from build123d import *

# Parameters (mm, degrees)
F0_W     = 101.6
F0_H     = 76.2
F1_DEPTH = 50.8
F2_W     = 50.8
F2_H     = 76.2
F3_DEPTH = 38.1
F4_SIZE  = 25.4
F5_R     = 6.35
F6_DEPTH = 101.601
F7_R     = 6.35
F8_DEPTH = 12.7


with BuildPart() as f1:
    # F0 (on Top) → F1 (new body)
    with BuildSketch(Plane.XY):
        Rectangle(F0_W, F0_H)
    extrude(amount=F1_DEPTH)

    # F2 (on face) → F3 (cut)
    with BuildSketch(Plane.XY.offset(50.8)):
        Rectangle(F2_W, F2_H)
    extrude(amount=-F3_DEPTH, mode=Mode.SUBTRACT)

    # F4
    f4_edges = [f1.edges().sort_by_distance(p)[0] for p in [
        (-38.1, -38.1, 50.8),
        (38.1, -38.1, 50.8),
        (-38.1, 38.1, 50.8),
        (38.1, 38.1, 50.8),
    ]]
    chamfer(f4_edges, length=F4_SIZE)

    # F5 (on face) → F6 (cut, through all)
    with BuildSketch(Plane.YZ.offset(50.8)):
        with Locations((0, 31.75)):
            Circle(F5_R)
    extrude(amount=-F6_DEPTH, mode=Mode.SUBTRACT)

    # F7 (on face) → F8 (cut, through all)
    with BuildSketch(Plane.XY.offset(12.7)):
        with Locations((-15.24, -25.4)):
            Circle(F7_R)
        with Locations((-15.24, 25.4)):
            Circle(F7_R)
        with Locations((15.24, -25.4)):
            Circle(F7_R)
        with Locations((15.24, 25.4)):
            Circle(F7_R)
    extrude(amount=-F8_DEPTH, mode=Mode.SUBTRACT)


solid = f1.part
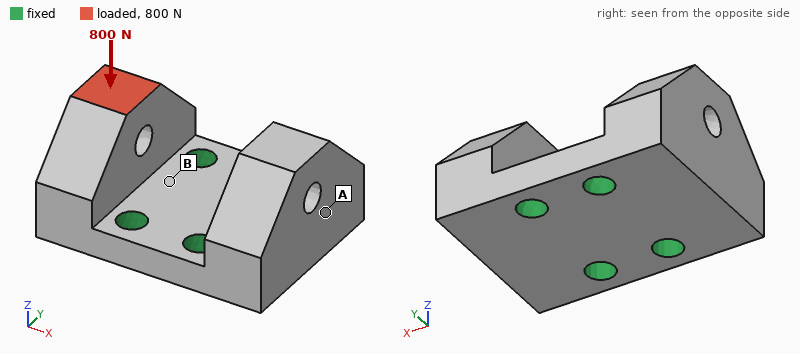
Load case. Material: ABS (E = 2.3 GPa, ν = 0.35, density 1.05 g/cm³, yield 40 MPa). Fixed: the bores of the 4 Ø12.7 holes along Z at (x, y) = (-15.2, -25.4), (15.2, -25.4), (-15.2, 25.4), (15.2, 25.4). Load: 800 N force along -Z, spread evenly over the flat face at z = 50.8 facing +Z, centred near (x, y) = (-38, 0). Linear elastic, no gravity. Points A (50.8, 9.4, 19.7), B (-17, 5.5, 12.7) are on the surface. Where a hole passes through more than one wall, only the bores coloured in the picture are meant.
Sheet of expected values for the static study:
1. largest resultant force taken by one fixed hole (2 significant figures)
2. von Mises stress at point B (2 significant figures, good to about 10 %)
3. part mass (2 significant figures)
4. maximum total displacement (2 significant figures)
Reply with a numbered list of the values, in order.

1. 440 N
2. 2.7 MPa
3. 210 g
4. 0.29 mm
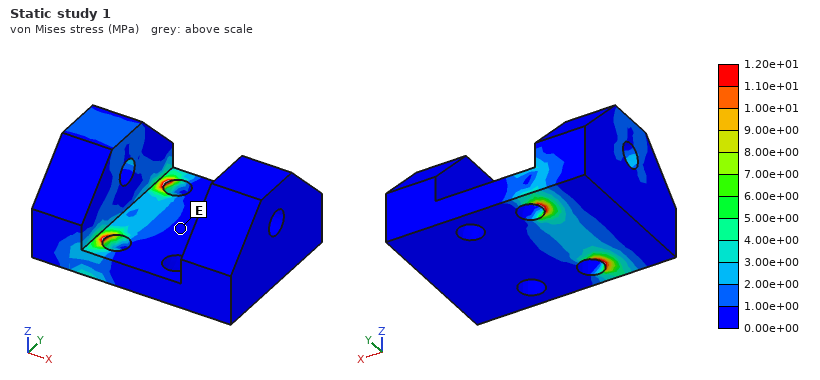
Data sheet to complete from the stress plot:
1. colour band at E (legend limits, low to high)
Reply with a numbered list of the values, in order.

1. 0.00e+00 to 1.00e+00 MPa
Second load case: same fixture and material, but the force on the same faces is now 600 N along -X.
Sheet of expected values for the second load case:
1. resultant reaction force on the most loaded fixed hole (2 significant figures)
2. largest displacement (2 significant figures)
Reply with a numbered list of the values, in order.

1. 280 N
2. 0.74 mm
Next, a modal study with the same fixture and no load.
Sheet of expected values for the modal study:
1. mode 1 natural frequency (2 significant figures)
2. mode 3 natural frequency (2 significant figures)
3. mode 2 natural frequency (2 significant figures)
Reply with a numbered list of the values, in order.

1. 980 Hz
2. 2300 Hz
3. 990 Hz
